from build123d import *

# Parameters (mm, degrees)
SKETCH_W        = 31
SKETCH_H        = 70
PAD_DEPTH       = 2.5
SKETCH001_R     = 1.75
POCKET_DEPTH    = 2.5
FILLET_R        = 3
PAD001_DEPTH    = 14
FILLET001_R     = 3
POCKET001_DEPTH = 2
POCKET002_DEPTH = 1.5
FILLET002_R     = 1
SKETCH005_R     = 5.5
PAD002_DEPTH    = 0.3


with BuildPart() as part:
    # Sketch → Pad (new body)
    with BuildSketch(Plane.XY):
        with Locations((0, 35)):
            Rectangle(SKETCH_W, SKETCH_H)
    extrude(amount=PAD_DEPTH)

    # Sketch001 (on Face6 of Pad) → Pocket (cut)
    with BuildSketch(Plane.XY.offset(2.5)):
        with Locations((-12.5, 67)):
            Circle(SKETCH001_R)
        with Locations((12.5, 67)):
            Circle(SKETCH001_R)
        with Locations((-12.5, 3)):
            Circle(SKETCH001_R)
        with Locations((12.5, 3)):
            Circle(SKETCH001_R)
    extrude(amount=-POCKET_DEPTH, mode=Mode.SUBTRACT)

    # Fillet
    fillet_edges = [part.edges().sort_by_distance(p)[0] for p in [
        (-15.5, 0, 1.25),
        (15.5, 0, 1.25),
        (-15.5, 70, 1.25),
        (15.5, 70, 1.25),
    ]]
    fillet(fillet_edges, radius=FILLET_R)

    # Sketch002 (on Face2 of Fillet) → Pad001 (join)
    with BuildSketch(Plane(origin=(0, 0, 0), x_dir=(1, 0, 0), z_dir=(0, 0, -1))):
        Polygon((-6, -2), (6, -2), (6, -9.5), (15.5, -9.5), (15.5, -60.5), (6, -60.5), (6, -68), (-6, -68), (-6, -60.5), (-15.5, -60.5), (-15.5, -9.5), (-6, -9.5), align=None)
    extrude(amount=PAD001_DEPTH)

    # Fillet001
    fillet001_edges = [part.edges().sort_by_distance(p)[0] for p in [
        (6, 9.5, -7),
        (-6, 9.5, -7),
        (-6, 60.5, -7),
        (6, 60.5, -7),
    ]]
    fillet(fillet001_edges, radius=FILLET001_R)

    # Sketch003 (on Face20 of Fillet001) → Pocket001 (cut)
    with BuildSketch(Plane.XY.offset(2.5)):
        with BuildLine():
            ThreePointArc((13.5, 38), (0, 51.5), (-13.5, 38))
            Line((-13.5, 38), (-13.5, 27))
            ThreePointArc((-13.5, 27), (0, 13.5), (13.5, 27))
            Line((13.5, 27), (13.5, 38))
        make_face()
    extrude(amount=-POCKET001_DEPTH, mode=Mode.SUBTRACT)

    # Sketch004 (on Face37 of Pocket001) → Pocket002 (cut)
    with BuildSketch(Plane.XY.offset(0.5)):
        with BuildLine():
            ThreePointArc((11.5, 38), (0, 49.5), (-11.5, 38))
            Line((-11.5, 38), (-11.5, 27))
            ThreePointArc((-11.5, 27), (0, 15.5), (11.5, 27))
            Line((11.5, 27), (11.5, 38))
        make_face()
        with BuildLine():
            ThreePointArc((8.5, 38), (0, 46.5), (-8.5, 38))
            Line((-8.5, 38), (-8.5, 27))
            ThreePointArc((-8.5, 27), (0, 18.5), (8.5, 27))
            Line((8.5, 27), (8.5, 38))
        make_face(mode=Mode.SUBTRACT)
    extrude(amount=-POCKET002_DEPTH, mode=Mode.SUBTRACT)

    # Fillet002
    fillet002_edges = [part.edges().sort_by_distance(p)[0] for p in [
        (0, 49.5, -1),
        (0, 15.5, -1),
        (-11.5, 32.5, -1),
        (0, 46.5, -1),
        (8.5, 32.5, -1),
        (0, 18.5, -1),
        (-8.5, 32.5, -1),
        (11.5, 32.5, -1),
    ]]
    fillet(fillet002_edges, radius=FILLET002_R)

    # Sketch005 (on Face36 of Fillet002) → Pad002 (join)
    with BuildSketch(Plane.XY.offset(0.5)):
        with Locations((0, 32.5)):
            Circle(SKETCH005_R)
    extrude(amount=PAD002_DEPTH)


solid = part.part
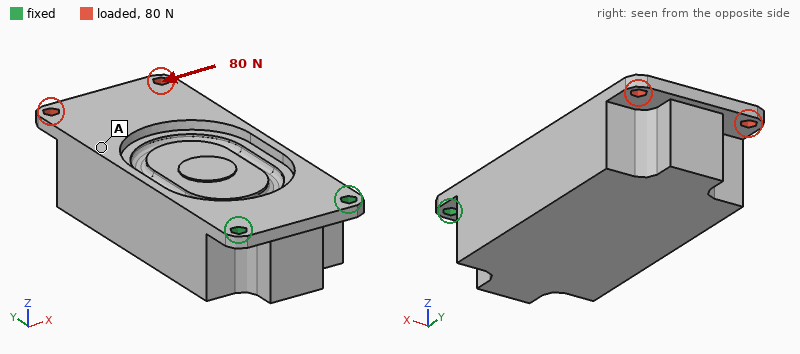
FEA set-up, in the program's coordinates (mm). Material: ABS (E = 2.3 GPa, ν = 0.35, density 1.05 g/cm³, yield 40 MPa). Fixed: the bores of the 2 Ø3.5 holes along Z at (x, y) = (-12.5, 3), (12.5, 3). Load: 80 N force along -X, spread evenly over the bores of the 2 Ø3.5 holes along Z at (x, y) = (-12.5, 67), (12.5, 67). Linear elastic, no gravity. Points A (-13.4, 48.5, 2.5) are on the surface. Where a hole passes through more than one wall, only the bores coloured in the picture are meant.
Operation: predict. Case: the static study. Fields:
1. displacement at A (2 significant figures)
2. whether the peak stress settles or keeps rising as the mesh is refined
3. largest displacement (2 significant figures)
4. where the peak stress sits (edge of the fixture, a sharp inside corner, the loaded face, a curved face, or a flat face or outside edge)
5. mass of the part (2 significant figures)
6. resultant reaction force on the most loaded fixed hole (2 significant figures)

0.26 mm
keeps rising
0.39 mm
edge of the fixture
29 g
200 N
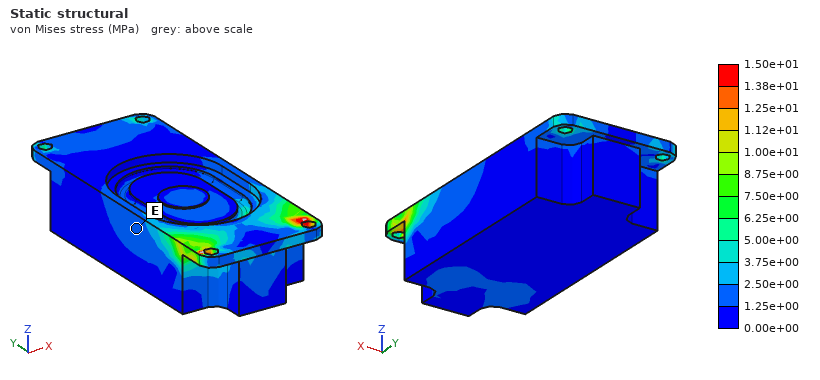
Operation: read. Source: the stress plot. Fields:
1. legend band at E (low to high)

1.25e+00 to 2.50e+00 MPa
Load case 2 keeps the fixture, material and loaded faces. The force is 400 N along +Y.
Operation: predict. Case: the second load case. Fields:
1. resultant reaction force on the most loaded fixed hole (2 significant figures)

200 N
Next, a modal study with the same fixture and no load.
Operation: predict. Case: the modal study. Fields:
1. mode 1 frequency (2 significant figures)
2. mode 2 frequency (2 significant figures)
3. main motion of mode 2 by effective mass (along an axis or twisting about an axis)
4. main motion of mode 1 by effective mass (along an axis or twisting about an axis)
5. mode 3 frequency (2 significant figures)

120 Hz
830 Hz
along X
along Z
1300 Hz
